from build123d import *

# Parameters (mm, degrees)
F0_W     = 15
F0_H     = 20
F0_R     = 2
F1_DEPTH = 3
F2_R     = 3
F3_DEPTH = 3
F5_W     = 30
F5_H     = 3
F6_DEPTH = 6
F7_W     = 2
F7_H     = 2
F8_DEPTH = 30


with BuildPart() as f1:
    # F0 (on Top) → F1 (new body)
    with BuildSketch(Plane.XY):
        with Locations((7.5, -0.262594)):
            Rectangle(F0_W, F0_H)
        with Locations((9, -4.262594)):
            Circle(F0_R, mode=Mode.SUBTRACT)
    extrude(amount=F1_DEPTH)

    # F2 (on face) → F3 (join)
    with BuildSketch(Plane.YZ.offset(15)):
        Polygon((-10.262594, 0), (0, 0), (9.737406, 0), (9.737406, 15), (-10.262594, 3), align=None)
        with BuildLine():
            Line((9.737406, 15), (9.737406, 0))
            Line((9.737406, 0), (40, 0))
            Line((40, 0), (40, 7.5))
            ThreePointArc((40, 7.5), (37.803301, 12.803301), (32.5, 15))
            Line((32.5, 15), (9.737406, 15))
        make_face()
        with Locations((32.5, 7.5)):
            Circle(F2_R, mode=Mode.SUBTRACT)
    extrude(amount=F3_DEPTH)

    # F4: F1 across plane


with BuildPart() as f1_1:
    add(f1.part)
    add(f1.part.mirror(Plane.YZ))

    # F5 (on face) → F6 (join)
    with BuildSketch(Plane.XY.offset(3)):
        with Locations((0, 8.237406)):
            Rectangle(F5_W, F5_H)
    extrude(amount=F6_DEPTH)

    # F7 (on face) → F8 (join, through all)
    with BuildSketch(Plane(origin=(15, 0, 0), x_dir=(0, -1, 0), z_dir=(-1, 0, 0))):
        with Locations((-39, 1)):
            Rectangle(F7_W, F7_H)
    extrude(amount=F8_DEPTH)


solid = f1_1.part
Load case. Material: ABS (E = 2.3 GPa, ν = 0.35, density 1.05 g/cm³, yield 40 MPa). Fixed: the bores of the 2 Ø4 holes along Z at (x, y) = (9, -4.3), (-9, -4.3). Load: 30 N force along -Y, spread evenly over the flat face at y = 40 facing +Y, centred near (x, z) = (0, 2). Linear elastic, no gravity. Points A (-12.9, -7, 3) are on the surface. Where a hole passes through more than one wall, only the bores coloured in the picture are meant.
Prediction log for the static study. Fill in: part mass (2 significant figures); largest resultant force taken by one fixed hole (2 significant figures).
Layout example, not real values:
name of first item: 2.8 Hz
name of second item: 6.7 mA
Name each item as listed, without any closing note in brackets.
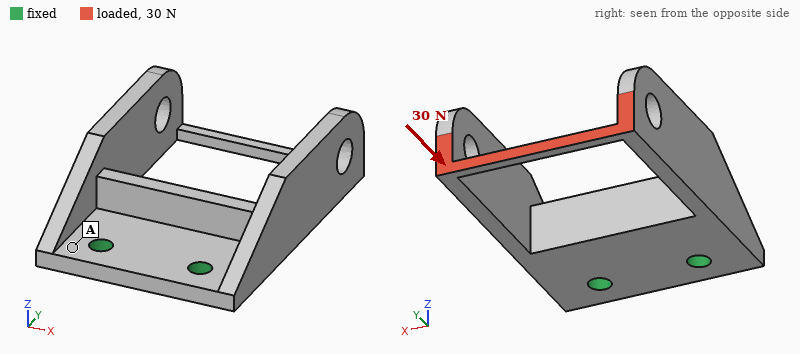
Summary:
part mass: 6.2 g
largest resultant force taken by one fixed hole: 16 N
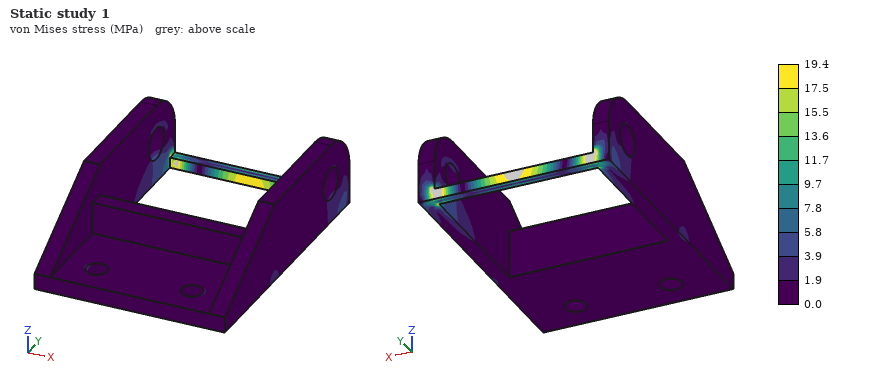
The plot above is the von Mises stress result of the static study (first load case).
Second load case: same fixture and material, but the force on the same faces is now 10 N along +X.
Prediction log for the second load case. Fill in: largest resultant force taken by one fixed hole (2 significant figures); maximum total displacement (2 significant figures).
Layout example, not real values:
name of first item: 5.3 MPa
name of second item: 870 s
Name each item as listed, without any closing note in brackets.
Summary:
largest resultant force taken by one fixed hole: 20 N
maximum total displacement: 0.72 mm
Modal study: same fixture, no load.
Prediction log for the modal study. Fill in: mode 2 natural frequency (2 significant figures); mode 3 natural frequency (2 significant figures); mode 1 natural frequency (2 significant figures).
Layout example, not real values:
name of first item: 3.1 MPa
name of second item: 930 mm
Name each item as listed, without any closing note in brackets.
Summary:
mode 2 natural frequency: 660 Hz
mode 3 natural frequency: 730 Hz
mode 1 natural frequency: 660 Hz
